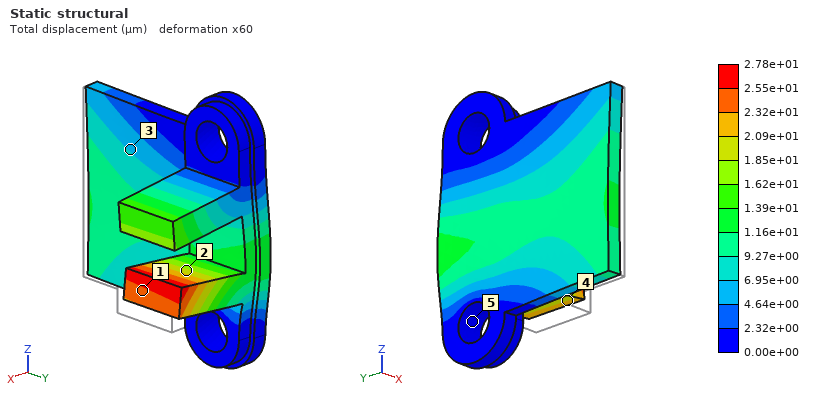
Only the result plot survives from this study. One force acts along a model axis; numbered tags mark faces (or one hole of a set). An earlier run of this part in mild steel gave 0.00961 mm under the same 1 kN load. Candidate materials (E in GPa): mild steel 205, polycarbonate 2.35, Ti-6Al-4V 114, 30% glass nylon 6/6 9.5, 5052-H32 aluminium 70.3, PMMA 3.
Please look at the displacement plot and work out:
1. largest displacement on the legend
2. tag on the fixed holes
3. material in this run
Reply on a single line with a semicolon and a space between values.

2.78e+01 µm; 5; 5052-H32 aluminium
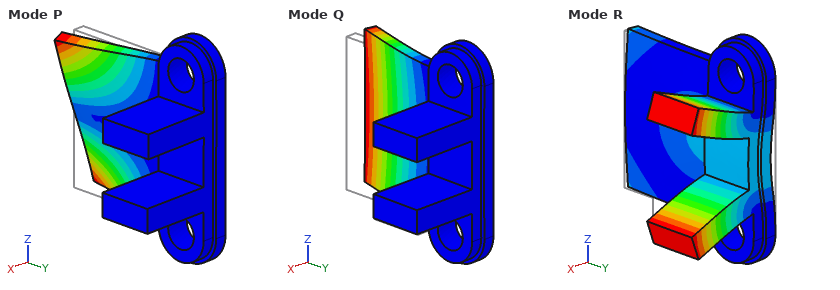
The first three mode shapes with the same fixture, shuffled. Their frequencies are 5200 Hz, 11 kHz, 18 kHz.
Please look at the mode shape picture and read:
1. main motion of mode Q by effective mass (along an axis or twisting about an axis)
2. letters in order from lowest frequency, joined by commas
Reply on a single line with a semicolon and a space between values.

along X; Q, P, R
